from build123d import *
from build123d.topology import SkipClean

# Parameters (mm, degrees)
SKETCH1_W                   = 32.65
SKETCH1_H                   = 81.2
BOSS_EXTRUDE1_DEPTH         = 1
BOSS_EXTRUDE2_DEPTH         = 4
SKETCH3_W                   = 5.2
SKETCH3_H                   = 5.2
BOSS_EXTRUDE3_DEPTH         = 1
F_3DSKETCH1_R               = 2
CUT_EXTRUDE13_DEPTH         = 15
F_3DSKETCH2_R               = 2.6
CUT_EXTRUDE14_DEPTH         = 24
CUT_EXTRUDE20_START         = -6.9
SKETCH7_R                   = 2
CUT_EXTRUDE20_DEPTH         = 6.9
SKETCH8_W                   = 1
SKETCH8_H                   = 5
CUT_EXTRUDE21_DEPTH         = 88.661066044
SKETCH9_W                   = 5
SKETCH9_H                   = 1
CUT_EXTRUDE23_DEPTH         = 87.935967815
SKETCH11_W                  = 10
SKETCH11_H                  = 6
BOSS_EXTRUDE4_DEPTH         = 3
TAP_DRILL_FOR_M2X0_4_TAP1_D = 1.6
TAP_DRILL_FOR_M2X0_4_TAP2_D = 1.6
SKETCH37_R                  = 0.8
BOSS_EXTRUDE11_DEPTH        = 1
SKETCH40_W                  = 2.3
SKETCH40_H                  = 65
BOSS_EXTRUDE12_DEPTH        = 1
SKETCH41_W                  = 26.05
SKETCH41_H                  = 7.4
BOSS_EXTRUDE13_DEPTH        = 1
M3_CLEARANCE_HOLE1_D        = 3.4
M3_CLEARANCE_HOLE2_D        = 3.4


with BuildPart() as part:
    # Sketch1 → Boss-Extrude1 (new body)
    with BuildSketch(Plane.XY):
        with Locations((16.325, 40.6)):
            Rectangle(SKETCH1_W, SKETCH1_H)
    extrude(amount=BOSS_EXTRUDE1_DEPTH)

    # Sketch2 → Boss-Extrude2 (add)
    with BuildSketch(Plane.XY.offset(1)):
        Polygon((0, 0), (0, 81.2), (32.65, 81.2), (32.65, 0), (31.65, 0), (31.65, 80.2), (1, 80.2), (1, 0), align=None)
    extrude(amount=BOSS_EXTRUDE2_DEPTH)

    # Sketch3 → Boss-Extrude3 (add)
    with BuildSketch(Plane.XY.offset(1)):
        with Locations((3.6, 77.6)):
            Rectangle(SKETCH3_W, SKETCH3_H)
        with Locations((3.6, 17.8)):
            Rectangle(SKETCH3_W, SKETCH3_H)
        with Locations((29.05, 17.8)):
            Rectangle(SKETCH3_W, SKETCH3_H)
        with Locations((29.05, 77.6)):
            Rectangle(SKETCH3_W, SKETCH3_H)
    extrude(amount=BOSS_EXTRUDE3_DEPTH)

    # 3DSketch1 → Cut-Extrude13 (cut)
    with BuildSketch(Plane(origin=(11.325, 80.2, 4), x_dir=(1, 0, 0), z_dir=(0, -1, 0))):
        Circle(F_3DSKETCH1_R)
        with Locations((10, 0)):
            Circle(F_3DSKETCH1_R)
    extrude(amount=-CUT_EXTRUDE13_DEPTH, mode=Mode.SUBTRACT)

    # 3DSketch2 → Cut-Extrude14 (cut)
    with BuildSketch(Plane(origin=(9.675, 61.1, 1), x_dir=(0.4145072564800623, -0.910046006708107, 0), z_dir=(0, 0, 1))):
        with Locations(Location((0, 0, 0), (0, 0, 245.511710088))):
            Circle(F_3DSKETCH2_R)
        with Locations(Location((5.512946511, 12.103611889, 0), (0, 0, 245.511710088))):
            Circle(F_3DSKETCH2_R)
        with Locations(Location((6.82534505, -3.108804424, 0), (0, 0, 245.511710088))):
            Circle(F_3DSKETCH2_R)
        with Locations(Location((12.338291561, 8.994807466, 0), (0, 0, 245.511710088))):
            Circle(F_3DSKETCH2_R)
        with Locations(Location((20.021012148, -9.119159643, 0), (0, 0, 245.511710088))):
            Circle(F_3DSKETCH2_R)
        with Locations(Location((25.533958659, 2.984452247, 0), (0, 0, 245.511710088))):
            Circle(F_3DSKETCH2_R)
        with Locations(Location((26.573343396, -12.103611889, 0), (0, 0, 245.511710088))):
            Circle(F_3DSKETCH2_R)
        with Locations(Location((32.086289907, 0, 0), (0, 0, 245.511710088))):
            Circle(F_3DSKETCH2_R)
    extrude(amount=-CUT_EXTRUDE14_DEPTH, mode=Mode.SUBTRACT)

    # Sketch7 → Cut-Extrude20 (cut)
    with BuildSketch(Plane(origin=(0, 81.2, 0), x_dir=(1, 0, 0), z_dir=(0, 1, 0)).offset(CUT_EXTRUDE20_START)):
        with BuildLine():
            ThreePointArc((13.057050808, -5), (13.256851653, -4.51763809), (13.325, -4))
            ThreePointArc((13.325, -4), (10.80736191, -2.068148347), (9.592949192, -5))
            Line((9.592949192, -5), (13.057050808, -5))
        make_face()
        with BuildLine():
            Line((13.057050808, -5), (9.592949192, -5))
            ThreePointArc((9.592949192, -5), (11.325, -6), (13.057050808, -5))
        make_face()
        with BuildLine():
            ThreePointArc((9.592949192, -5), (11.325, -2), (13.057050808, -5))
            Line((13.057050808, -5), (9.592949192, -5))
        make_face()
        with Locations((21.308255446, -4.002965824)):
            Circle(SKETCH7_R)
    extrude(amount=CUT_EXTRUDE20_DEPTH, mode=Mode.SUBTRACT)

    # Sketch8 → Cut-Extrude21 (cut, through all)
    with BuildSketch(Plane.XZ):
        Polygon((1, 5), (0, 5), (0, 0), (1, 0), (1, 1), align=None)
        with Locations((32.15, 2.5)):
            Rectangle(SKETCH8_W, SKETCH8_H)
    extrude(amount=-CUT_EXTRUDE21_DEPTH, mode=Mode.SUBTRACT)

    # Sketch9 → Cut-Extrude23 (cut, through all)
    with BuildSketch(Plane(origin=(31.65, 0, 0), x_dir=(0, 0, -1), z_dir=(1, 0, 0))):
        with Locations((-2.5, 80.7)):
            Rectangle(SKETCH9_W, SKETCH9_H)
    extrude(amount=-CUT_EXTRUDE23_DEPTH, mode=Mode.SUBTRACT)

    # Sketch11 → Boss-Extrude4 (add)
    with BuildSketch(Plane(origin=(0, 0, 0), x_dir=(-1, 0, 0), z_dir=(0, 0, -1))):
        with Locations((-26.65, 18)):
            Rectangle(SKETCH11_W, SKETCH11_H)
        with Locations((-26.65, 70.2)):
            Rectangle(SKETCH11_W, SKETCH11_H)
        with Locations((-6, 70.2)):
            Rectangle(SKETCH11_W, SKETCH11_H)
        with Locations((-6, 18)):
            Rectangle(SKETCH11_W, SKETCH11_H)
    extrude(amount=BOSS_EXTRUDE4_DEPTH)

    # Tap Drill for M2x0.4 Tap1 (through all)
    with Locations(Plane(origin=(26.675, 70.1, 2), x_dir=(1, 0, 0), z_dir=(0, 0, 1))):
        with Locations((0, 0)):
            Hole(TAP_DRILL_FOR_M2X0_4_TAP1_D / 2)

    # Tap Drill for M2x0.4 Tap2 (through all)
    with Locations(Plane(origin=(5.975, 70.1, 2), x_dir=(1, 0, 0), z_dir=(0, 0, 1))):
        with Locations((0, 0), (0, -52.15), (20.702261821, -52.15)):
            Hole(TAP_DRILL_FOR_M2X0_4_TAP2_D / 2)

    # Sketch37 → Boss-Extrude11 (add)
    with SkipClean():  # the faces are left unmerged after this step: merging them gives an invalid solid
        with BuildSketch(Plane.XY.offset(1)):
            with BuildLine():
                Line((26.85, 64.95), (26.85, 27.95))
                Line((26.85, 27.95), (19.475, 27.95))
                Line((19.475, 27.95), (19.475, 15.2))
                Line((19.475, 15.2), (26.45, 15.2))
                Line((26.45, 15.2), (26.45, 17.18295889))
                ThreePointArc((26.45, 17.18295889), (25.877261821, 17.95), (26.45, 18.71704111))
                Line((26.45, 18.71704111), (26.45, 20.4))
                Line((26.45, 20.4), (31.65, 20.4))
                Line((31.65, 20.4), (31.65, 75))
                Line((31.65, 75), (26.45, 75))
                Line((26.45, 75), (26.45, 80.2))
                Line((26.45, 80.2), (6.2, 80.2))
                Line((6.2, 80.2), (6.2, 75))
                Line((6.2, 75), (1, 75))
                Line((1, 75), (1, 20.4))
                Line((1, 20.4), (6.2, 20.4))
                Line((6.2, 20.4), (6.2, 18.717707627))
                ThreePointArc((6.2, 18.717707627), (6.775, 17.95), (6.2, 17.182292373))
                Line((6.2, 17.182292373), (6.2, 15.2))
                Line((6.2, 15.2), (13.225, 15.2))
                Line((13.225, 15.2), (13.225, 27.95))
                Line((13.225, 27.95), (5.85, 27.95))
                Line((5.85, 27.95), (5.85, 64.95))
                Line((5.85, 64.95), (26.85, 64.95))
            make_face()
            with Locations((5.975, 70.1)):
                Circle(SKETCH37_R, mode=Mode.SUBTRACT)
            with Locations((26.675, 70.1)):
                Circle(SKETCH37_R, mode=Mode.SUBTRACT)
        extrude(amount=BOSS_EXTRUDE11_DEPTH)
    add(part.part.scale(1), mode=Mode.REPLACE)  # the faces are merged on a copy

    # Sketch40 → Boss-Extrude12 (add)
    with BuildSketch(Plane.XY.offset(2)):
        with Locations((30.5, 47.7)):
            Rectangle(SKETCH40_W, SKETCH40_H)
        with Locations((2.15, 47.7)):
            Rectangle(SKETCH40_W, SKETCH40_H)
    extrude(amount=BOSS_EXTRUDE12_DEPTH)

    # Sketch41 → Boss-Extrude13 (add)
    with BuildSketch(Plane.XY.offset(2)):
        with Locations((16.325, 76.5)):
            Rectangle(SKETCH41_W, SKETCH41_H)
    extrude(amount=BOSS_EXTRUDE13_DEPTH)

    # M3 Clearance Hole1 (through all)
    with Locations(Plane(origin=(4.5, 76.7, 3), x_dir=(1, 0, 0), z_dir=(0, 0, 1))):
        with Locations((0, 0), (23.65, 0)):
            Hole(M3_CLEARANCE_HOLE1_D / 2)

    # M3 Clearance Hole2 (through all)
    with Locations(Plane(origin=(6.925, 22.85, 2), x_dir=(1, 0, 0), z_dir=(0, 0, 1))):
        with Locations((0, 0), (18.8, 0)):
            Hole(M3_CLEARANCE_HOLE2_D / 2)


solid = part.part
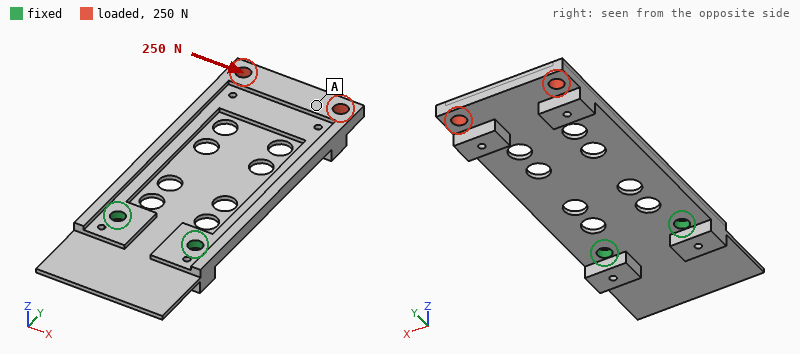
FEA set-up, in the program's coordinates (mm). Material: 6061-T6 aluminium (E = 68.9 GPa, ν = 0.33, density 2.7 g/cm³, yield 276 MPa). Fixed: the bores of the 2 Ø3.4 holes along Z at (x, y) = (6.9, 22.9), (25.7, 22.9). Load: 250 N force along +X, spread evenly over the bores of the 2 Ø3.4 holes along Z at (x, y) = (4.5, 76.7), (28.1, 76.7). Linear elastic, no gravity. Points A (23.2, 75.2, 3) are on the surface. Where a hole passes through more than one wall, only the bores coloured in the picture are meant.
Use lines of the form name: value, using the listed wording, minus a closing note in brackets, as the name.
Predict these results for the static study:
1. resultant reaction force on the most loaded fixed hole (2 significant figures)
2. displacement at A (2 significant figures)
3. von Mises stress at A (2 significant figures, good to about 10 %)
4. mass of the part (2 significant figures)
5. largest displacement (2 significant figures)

resultant reaction force on the most loaded fixed hole: 640 N
displacement at A: 0.12 mm
von Mises stress at A: 9.8 MPa
mass of the part: 12 g
largest displacement: 0.19 mm
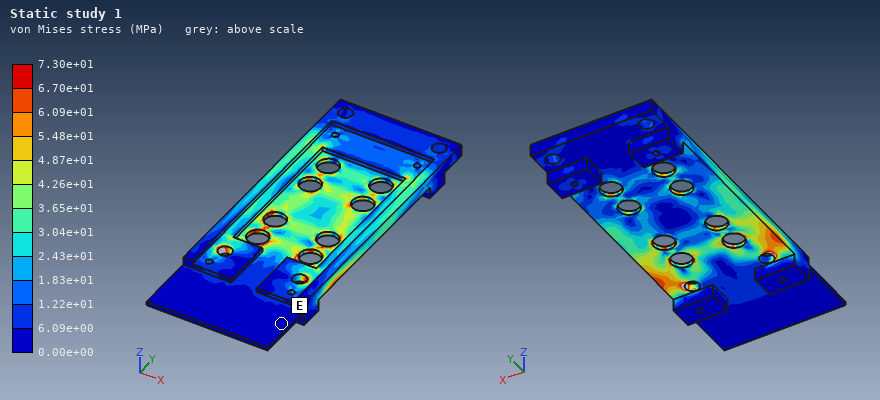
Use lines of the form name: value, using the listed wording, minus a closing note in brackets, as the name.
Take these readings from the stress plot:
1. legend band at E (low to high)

legend band at E: 0.00e+00 to 6.09e+00 MPa
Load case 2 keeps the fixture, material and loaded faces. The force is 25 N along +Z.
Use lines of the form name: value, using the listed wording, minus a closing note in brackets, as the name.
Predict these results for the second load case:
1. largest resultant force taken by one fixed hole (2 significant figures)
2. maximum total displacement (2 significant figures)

largest resultant force taken by one fixed hole: 25 N
maximum total displacement: 0.96 mm
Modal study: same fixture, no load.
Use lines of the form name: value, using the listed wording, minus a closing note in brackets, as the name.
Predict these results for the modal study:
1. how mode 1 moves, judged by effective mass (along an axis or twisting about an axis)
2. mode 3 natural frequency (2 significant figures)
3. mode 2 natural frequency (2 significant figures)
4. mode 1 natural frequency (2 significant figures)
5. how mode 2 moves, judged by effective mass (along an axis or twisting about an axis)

how mode 1 moves, judged by effective mass: along Z
mode 3 natural frequency: 3200 Hz
mode 2 natural frequency: 1400 Hz
mode 1 natural frequency: 440 Hz
how mode 2 moves, judged by effective mass: twisting about Y
